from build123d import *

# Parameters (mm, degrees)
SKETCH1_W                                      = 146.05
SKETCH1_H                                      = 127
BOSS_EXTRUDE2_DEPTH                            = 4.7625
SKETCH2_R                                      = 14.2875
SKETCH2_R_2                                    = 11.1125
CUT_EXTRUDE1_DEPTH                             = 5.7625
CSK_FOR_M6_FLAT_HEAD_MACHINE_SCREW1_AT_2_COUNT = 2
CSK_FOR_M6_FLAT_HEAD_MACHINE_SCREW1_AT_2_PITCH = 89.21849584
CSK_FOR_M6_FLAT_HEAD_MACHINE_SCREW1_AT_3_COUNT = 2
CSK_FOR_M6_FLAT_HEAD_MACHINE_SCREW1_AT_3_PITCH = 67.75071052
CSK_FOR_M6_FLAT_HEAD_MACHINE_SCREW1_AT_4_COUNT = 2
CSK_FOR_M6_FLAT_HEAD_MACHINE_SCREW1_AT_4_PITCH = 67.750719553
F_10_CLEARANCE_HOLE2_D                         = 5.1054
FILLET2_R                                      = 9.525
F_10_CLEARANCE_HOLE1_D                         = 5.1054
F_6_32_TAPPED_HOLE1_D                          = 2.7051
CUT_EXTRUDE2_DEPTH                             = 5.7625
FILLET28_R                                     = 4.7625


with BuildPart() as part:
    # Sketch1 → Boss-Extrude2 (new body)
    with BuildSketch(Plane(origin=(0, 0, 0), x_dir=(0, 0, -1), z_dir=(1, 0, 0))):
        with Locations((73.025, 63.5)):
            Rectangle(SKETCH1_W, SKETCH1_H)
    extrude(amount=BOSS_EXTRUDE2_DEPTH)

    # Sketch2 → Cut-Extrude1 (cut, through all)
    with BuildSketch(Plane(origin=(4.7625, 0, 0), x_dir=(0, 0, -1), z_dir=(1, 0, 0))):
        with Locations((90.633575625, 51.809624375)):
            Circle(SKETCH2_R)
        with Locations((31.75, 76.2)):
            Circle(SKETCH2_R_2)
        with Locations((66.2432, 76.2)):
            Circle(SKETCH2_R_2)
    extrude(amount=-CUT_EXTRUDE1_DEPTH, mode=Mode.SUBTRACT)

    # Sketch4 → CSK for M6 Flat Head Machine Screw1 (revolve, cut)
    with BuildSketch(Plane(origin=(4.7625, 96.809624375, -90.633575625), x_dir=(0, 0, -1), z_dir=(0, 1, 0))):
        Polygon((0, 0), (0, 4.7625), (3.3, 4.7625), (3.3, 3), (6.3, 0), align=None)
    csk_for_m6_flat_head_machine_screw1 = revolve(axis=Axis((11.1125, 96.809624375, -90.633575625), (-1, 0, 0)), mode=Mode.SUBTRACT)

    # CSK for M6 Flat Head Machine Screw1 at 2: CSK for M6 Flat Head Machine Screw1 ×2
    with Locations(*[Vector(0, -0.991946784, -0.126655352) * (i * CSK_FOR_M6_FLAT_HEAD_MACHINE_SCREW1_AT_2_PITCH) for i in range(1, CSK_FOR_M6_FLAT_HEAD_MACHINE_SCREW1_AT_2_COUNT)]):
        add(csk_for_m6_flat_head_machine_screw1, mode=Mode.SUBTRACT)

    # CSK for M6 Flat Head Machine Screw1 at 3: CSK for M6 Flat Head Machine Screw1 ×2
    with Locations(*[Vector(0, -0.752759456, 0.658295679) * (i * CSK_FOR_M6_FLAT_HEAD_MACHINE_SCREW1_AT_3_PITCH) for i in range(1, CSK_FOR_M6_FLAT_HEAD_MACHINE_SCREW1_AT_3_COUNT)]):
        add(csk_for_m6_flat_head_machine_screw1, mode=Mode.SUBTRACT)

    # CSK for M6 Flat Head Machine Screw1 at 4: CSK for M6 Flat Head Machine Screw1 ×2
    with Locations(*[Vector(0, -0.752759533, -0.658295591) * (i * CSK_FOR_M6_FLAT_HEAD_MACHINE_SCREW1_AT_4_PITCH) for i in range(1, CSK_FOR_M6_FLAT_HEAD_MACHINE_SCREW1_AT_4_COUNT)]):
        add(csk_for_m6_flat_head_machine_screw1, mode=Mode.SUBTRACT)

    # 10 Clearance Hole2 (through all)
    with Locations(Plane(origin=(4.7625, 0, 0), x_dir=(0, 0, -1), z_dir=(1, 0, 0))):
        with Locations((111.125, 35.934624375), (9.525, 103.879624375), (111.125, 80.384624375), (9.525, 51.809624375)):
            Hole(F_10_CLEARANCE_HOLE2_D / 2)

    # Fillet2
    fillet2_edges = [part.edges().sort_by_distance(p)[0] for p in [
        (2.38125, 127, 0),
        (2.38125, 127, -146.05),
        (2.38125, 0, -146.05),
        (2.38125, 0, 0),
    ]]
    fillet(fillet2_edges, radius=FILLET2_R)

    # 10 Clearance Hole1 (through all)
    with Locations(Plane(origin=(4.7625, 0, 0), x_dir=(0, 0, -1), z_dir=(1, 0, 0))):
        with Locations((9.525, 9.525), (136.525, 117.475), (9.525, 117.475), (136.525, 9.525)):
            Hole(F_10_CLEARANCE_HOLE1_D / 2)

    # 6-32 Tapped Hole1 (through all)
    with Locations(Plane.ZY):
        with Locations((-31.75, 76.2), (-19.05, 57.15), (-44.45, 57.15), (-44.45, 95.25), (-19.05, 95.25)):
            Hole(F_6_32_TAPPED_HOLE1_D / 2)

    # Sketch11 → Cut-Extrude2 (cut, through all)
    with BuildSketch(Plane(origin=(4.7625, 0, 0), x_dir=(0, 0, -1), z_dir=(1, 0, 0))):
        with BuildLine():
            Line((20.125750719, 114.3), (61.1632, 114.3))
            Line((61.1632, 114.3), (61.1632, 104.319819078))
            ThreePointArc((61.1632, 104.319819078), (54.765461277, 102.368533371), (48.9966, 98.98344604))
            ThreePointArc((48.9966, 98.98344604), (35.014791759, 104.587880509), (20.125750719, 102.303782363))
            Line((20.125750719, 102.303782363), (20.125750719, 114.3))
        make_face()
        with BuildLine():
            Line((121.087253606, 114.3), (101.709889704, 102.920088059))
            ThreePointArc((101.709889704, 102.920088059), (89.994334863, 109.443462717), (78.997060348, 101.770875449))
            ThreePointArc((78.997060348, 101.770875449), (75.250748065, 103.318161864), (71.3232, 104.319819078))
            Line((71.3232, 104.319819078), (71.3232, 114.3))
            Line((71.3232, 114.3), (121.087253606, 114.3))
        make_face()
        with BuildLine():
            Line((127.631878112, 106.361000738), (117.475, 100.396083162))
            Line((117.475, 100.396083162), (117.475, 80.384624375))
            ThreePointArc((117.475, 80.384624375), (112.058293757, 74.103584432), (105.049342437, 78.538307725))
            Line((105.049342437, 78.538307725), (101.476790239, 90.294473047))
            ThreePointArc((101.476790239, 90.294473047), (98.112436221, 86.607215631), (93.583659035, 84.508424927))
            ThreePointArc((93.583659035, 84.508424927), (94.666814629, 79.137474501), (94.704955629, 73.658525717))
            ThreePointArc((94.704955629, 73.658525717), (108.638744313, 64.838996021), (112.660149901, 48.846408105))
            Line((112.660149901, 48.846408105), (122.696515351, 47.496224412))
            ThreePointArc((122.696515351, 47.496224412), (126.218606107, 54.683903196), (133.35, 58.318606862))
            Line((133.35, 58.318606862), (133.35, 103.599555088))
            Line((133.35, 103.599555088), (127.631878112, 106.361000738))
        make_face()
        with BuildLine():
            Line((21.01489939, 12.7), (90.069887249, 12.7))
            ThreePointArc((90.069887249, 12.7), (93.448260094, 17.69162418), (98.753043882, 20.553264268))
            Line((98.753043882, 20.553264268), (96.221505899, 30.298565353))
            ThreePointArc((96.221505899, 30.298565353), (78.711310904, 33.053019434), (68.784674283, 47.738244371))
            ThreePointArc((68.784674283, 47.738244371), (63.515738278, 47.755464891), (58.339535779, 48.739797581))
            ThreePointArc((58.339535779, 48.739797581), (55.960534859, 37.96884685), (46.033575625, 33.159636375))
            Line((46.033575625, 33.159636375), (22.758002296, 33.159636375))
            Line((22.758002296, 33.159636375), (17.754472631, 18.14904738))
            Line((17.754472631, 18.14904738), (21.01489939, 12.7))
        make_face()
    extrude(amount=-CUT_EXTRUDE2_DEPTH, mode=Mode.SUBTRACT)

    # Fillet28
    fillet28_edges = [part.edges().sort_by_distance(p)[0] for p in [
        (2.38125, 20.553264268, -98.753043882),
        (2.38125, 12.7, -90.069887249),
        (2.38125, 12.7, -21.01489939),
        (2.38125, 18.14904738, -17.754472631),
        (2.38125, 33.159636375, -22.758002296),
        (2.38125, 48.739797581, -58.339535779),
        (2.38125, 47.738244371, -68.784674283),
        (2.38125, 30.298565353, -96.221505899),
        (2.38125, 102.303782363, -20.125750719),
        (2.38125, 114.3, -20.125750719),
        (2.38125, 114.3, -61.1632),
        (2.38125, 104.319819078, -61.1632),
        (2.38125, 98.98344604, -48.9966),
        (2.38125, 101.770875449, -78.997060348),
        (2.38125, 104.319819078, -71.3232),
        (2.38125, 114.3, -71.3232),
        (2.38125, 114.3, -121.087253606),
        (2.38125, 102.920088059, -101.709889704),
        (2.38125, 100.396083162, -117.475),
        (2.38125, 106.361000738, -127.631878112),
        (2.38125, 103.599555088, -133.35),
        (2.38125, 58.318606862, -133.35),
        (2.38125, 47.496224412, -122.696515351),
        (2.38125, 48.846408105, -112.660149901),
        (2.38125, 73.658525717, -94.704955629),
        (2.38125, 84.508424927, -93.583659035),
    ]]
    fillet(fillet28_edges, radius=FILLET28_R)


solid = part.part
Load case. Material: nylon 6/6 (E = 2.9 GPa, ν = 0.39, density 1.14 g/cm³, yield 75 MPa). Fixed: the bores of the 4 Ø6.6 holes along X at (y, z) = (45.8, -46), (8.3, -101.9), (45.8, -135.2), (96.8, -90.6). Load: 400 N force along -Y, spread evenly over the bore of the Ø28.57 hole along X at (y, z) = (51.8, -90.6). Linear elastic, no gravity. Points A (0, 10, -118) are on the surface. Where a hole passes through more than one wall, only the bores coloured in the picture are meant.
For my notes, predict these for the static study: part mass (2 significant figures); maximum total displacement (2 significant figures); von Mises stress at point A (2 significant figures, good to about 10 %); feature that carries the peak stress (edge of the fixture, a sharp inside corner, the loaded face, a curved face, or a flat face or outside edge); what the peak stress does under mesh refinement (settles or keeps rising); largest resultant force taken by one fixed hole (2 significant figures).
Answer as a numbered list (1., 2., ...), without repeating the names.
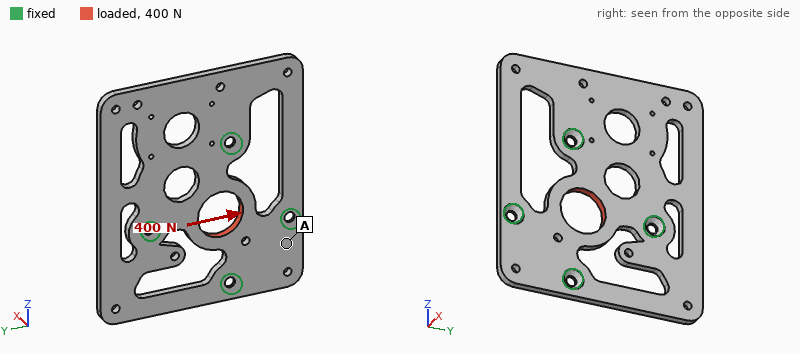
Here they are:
1. 71 g
2. 57 µm
3. 0.41 MPa
4. edge of the fixture
5. keeps rising
6. 140 N
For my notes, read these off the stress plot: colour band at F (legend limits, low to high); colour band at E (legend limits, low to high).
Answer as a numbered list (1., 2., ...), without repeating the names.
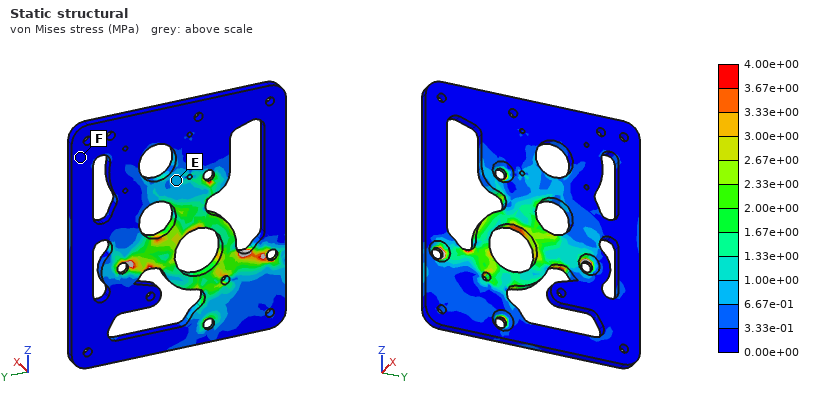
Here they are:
1. 0.00e+00 to 3.33e-01 MPa
2. 6.67e-01 to 1.00e+00 MPa
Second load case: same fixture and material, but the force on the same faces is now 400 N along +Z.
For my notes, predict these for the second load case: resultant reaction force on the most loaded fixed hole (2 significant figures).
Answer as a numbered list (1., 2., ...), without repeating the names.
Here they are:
1. 130 N
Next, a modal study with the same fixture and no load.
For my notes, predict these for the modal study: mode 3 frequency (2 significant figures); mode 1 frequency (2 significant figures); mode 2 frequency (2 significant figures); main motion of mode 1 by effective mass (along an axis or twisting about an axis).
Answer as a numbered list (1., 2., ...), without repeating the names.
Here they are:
1. 360 Hz
2. 210 Hz
3. 320 Hz
4. along X
